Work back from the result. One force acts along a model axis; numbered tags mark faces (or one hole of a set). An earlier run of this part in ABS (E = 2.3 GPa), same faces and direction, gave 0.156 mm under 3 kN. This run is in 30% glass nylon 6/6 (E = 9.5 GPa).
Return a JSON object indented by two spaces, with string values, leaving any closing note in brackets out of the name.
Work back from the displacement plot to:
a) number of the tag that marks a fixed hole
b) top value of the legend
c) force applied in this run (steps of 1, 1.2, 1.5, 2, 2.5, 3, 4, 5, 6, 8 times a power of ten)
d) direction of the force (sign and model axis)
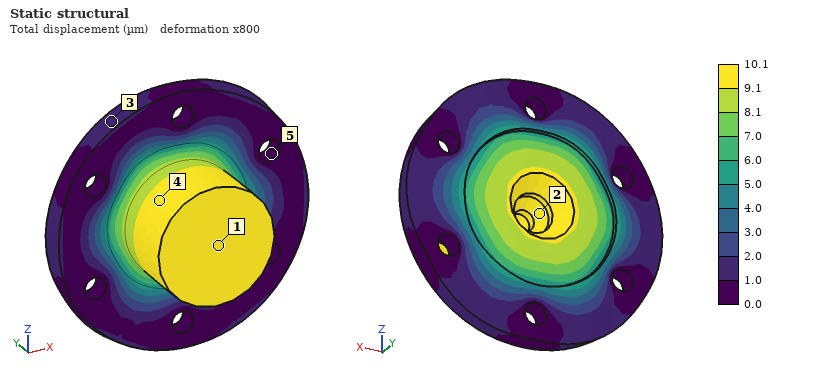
{
  "number of the tag that marks a fixed hole": "5",
  "top value of the legend": "10.1 µm",
  "force applied in this run": "800 N",
  "direction of the force": "+Y"
}
